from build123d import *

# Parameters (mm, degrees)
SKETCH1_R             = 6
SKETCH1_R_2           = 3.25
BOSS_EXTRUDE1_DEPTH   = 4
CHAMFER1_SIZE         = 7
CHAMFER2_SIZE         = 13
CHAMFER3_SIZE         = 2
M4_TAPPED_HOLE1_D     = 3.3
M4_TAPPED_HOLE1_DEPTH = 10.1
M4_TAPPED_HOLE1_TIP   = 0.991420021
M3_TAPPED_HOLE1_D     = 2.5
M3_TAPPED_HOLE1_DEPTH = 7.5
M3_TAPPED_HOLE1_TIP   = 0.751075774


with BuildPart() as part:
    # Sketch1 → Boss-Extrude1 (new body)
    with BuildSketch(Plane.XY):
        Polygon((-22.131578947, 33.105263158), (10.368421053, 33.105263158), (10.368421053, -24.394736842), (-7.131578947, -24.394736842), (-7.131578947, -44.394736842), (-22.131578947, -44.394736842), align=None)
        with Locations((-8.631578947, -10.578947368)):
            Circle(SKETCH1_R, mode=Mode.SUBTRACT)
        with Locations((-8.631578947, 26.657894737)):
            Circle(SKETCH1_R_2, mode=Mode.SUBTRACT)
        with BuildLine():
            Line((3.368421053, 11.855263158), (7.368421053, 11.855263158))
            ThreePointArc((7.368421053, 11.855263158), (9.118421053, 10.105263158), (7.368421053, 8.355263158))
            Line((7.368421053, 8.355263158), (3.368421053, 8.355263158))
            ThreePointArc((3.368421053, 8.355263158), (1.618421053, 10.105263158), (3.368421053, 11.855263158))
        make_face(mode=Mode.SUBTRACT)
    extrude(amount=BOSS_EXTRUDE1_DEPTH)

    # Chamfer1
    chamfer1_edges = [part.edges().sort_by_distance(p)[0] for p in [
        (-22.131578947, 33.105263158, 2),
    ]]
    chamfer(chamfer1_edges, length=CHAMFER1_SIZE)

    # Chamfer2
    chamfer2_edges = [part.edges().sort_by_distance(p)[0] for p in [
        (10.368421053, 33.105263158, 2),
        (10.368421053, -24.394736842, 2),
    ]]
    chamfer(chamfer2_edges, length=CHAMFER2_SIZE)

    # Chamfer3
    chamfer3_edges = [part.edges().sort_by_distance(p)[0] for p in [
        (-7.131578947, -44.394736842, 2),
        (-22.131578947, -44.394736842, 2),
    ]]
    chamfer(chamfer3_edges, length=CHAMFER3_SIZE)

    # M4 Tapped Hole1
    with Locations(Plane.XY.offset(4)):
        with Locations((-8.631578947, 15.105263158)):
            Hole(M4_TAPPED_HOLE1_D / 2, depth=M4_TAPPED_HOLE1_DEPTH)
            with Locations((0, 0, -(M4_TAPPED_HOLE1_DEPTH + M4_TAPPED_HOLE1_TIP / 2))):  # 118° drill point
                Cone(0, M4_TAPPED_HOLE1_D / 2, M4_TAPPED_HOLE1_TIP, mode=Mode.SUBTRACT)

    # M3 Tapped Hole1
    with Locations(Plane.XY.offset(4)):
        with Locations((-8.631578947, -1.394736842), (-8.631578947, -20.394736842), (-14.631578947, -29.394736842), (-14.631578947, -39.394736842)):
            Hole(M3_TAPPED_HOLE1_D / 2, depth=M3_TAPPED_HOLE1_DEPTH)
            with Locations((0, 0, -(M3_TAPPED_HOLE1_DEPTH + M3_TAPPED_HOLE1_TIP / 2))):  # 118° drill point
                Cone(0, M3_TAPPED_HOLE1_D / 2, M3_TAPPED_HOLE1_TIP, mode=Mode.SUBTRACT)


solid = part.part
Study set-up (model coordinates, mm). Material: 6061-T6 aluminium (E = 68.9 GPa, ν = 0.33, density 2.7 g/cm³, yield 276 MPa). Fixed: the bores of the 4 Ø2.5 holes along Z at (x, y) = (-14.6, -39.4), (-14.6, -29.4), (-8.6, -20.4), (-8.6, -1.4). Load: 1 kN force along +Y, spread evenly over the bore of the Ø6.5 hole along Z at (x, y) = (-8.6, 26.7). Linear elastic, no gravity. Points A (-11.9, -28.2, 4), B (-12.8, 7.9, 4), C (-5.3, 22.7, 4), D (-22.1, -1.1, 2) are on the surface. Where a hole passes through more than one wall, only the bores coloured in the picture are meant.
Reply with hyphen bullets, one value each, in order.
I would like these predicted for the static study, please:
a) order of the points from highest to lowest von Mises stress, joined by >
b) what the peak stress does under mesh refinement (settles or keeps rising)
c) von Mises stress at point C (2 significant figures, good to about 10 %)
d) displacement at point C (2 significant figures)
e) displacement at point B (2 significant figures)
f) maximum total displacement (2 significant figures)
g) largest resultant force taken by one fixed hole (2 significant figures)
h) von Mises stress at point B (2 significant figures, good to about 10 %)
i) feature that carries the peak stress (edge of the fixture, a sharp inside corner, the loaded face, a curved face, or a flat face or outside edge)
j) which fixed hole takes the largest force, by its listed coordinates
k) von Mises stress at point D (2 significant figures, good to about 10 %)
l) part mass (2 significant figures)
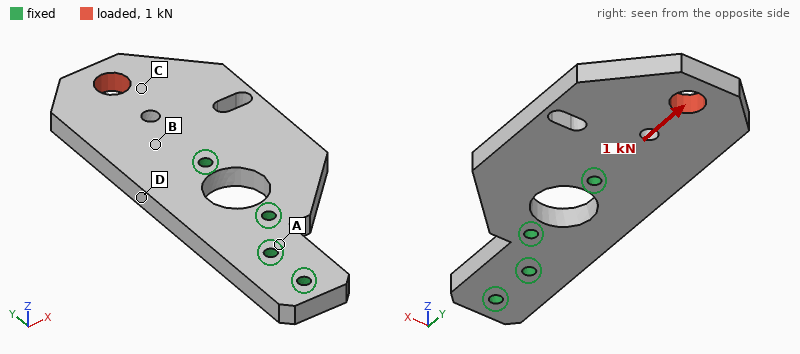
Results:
- C > B > D > A
- keeps rising
- 19 MPa
- 5.5 µm
- 2.5 µm
- 8.8 µm
- 740 N
- 12 MPa
- edge of the fixture
- (-8.6, -1.4)
- 7.3 MPa
- 19 g
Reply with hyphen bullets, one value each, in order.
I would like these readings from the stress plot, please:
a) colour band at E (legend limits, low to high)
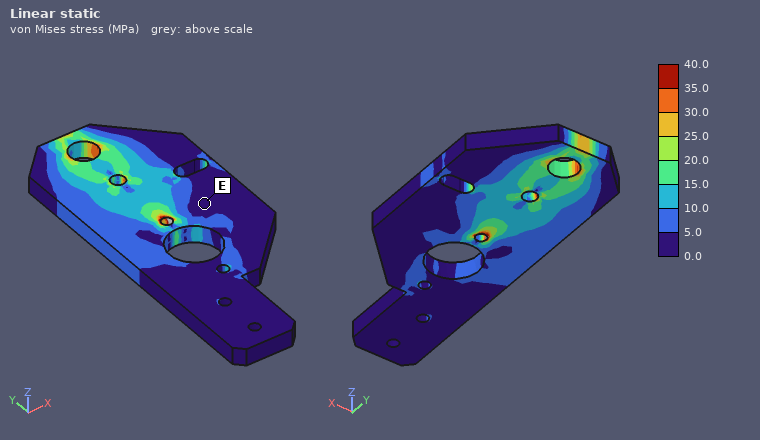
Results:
- 0.0 to 5.0 MPa
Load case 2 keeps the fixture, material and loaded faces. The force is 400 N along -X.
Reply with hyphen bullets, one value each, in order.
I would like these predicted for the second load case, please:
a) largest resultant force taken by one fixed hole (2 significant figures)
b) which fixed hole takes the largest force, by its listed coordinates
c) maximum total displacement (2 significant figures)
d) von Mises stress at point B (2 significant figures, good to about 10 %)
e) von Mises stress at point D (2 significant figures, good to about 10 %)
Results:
- 770 N
- (-8.6, -1.4)
- 28 µm
- 7.2 MPa
- 25 MPa
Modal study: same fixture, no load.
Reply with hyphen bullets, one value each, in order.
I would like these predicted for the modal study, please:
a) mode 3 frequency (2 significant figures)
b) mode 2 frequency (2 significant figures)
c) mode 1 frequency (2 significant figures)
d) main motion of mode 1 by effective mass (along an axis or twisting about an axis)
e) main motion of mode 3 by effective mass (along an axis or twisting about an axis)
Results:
- 9500 Hz
- 5100 Hz
- 2800 Hz
- along Z
- along X
